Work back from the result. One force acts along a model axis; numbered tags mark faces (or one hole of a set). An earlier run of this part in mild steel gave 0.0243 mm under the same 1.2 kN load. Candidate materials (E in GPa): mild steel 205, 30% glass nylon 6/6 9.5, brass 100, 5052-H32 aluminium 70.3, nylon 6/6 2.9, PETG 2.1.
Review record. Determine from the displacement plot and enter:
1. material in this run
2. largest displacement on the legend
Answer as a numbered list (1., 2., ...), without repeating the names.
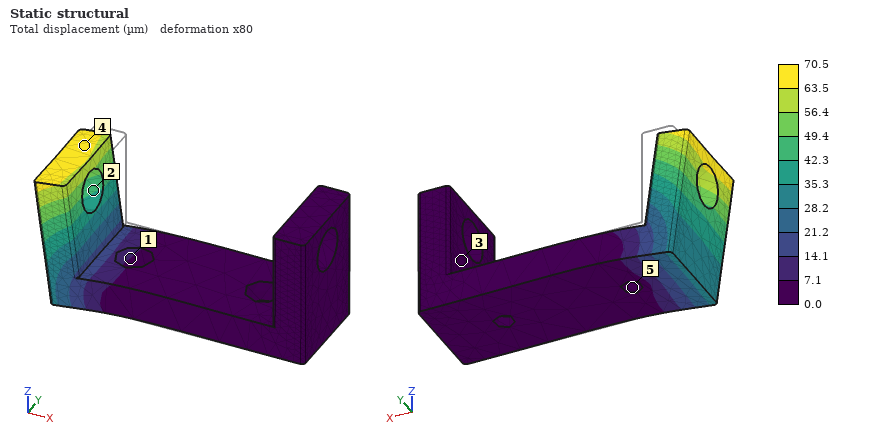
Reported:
1. 5052-H32 aluminium
2. 70.5 µm
